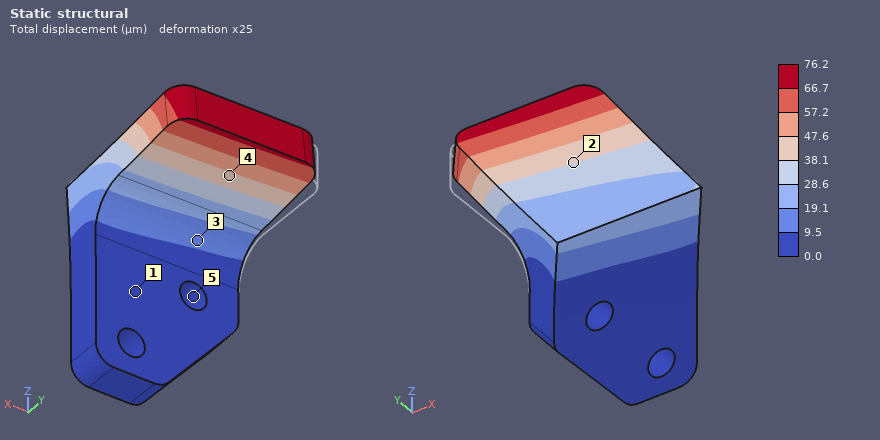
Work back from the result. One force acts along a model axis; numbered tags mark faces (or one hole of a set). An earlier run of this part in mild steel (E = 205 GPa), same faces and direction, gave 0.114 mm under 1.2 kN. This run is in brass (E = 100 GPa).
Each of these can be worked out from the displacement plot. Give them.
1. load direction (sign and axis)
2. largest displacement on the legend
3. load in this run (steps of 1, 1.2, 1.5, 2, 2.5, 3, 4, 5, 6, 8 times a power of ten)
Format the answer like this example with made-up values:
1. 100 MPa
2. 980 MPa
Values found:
1. +Z
2. 76.2 µm
3. 400 N
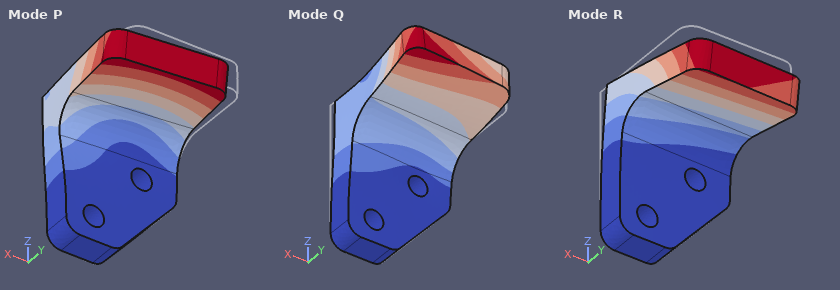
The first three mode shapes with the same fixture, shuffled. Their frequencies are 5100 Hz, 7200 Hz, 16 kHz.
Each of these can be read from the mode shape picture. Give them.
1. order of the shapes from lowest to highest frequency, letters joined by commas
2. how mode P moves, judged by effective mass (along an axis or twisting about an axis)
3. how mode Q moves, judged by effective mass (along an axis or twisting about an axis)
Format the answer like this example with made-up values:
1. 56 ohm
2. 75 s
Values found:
1. R, P, Q
2. along X
3. along Y
